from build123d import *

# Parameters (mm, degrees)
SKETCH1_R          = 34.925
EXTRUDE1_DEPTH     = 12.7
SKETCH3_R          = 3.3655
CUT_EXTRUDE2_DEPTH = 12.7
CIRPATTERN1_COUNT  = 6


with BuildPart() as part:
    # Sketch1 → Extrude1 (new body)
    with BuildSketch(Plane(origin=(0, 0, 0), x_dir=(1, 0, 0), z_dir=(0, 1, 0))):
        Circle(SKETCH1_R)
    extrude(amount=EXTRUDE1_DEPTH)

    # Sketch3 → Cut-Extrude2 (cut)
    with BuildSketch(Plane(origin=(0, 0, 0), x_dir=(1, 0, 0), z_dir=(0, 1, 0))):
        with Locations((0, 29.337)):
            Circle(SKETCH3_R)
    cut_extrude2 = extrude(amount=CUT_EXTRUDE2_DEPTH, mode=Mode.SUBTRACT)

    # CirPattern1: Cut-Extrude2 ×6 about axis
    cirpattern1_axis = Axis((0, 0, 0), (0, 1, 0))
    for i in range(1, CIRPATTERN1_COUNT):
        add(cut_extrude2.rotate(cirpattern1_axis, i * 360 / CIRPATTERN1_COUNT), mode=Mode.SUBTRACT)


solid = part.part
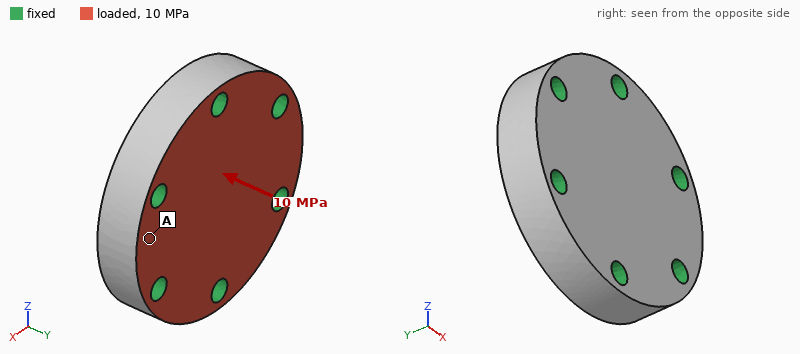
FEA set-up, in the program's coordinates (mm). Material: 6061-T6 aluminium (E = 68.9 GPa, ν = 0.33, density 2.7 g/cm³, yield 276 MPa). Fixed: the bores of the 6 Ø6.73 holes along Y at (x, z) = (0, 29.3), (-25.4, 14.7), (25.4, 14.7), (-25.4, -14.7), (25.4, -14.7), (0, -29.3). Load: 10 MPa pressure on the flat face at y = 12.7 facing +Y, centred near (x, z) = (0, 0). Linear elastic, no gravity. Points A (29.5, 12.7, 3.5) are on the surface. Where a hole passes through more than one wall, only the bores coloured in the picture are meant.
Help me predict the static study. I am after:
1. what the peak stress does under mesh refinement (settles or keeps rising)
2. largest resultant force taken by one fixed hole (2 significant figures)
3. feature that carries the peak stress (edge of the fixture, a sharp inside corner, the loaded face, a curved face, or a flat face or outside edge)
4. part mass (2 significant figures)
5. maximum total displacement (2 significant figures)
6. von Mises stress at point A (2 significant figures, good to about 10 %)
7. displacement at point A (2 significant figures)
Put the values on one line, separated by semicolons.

keeps rising; 6.1 kN; edge of the fixture; 120 g; 18 µm; 17 MPa; 5.2 µm
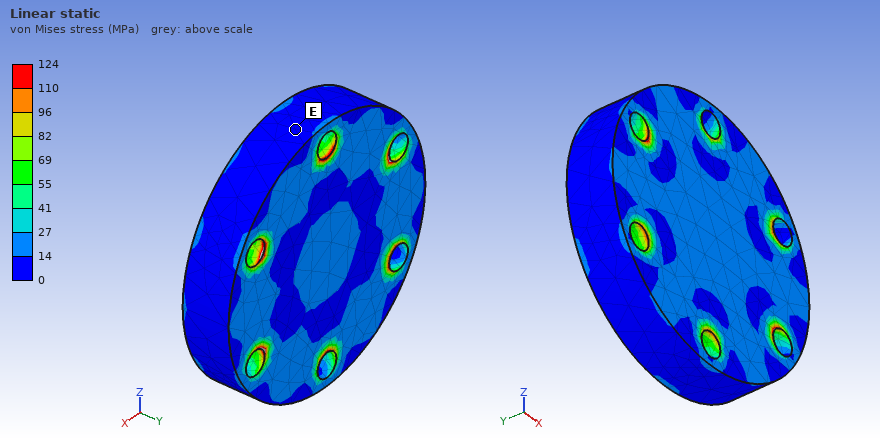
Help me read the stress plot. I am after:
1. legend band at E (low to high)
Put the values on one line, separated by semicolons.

0 to 14 MPa
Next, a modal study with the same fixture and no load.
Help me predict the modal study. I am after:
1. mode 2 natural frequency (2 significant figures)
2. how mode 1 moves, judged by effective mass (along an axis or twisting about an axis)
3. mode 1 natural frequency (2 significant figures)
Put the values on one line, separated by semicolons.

41 kHz; along Y; 24 kHz
